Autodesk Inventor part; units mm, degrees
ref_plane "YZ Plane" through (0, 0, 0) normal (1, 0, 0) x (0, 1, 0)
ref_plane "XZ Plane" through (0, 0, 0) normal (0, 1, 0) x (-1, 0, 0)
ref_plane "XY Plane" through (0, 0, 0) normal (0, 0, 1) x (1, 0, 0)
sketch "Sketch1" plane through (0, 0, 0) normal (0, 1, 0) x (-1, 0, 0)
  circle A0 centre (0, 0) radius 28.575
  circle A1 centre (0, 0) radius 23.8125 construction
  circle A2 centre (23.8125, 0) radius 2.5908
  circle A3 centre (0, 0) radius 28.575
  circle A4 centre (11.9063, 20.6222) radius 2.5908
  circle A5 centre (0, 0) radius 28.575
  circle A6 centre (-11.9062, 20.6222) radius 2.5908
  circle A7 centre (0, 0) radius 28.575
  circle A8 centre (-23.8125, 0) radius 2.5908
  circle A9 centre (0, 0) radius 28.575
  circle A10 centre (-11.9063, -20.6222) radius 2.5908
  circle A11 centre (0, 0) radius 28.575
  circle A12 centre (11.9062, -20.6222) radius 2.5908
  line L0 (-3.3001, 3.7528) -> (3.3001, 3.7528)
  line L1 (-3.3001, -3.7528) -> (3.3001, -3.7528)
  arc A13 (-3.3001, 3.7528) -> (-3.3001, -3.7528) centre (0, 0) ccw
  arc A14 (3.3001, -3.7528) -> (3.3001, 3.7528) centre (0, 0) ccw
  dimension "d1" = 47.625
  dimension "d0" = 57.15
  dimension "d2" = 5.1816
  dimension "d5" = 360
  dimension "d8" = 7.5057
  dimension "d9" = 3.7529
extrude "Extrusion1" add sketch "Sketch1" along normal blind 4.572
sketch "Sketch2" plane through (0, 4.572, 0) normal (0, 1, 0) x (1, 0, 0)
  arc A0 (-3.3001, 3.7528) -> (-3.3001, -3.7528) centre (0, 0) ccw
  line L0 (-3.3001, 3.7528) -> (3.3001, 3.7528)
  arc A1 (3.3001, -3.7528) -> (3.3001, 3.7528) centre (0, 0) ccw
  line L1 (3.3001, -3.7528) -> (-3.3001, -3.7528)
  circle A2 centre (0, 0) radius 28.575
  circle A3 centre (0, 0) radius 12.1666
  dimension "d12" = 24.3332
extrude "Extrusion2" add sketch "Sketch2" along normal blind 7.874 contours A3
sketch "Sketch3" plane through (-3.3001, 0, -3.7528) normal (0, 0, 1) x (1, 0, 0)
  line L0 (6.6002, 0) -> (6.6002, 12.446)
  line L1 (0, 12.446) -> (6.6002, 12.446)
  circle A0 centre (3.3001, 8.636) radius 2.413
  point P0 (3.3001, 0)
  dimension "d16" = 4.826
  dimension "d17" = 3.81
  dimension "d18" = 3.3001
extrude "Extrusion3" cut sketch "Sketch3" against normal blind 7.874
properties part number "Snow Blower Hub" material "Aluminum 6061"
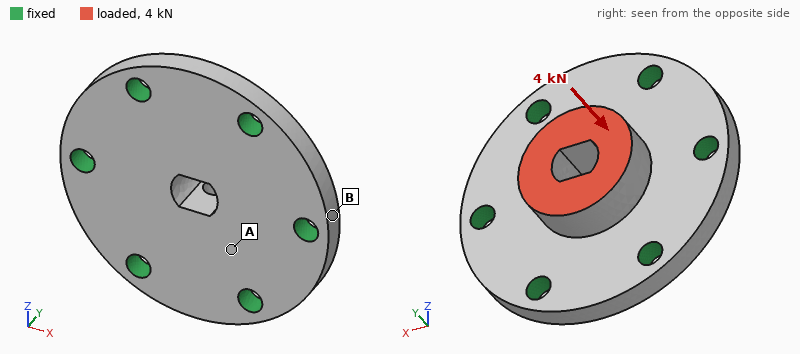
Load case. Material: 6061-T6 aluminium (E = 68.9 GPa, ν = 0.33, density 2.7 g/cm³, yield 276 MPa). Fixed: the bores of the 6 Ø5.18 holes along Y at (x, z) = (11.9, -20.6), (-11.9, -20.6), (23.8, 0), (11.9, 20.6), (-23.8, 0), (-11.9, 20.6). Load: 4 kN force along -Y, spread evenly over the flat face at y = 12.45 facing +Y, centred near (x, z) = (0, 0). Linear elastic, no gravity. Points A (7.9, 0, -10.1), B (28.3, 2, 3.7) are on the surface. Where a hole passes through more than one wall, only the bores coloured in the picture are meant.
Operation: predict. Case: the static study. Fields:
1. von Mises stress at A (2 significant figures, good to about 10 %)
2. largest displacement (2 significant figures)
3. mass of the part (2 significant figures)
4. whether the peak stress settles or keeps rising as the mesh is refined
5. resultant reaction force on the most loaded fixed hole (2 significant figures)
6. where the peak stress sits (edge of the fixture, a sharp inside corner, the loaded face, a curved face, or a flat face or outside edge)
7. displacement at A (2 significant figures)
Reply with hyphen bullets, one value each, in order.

- 31 MPa
- 23 µm
- 37 g
- keeps rising
- 740 N
- edge of the fixture
- 17 µm
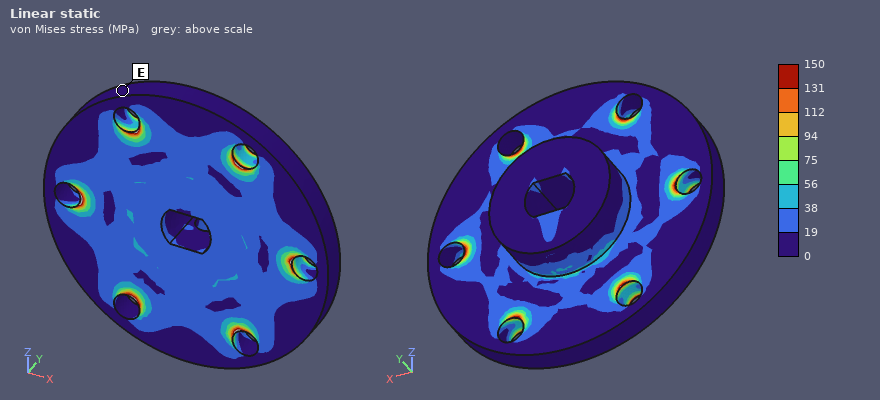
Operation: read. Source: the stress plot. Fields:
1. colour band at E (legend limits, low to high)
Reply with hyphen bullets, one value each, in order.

- 0 to 19 MPa
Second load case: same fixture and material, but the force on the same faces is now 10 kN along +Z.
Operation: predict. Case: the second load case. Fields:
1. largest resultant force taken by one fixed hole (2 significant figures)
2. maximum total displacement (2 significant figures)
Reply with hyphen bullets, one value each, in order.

- 2.7 kN
- 67 µm
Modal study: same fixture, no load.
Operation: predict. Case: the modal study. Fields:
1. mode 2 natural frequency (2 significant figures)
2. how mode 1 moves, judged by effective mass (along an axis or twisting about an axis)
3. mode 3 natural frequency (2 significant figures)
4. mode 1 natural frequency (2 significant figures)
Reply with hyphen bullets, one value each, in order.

- 26 kHz
- along Y
- 26 kHz
- 17 kHz
